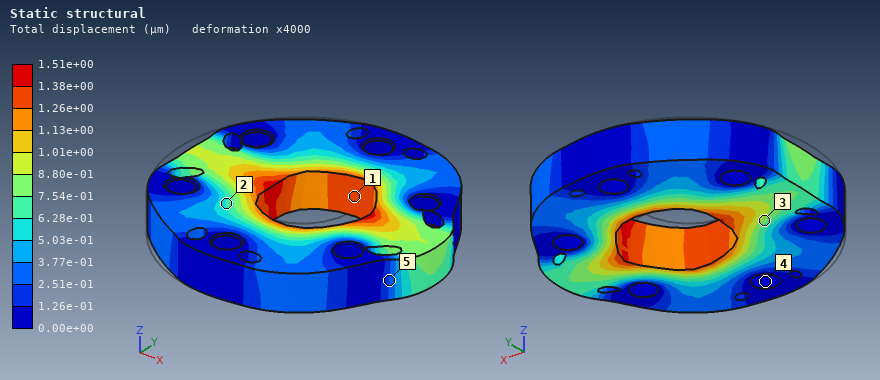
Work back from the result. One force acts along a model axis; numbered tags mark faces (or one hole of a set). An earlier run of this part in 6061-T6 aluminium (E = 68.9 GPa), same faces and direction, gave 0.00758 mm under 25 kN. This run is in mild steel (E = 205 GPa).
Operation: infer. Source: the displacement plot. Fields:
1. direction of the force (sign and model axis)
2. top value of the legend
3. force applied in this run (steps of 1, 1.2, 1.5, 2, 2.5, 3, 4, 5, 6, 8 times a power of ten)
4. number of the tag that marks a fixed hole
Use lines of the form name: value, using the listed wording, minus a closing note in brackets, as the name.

direction of the force: +X
top value of the legend: 1.51e+00 µm
force applied in this run: 15 kN
number of the tag that marks a fixed hole: 4
